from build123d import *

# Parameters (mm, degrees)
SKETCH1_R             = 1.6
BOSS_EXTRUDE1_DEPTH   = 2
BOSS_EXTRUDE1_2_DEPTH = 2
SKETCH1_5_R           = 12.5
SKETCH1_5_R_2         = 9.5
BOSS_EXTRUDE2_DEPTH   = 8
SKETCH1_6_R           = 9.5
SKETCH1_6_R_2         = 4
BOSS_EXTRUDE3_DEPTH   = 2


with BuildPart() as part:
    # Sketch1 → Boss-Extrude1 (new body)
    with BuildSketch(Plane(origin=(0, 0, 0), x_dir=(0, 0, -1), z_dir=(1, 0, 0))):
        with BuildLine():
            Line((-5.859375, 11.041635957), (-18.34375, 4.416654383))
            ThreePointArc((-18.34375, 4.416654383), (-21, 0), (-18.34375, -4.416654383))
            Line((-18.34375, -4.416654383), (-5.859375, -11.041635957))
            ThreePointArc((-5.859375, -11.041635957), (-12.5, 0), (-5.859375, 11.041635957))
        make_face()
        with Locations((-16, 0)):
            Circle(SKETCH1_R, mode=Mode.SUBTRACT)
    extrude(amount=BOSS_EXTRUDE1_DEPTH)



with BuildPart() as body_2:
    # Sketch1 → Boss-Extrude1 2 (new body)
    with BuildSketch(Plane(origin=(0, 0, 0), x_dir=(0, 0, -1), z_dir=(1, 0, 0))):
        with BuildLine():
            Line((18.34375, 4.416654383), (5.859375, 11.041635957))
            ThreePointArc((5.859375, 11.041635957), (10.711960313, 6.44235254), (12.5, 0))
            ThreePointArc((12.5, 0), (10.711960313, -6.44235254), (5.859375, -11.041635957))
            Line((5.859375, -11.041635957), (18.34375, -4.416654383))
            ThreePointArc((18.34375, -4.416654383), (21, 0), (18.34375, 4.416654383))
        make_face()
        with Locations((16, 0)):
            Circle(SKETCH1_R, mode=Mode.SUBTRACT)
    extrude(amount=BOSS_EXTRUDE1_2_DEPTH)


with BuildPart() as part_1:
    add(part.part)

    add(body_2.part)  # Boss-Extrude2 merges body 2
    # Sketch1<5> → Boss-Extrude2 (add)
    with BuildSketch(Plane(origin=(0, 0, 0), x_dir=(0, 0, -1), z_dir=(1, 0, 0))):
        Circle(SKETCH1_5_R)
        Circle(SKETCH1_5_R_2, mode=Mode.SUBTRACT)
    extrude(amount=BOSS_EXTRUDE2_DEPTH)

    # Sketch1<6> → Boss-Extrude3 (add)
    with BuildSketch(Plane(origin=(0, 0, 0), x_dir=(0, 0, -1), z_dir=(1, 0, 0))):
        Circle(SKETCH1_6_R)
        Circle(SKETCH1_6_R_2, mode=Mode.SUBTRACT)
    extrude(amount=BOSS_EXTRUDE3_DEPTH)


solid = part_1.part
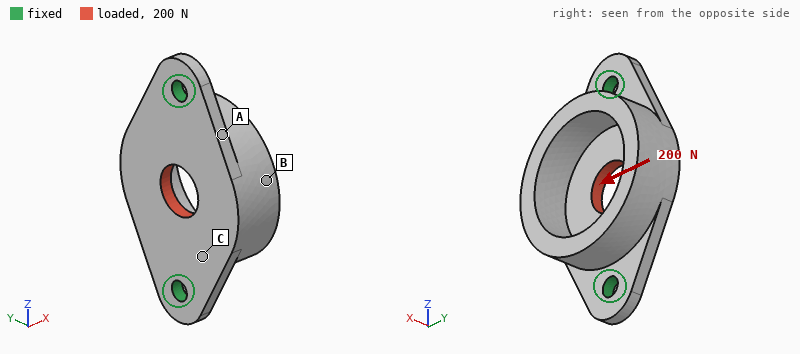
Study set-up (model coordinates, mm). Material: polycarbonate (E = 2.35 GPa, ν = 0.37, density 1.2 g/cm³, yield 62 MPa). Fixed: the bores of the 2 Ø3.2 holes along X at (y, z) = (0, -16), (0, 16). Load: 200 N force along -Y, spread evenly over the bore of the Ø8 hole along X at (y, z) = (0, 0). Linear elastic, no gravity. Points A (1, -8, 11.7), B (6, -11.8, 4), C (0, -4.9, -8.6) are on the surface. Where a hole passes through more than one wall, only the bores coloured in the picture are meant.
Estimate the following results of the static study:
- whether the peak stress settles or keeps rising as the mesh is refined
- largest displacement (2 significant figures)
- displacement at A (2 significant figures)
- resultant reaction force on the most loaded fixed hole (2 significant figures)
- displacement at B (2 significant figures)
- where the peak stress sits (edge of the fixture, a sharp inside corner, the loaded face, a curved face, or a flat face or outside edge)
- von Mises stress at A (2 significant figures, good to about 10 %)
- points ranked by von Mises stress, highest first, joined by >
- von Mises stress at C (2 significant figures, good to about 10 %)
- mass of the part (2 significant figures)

keeps rising
60 µm
29 µm
100 N
32 µm
edge of the fixture
5.6 MPa
A > C > B
3.3 MPa
3.0 g
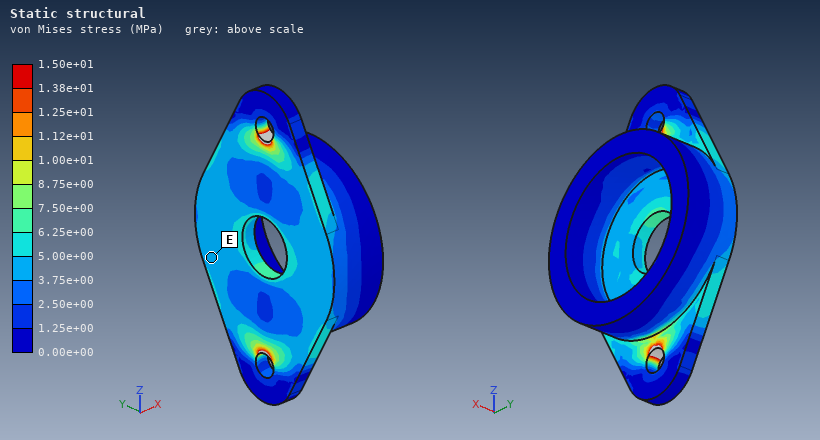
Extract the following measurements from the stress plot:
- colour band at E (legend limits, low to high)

3.75e+00 to 5.00e+00 MPa
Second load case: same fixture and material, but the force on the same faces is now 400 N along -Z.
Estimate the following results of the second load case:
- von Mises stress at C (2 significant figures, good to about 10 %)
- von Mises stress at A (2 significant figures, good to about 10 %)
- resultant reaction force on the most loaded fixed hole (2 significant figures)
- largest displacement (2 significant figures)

5.9 MPa
2.0 MPa
200 N
56 µm
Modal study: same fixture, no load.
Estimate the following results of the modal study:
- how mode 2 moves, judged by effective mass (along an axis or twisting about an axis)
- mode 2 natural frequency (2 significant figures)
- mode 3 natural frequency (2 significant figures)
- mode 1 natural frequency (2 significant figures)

along X
3100 Hz
6600 Hz
1700 Hz
